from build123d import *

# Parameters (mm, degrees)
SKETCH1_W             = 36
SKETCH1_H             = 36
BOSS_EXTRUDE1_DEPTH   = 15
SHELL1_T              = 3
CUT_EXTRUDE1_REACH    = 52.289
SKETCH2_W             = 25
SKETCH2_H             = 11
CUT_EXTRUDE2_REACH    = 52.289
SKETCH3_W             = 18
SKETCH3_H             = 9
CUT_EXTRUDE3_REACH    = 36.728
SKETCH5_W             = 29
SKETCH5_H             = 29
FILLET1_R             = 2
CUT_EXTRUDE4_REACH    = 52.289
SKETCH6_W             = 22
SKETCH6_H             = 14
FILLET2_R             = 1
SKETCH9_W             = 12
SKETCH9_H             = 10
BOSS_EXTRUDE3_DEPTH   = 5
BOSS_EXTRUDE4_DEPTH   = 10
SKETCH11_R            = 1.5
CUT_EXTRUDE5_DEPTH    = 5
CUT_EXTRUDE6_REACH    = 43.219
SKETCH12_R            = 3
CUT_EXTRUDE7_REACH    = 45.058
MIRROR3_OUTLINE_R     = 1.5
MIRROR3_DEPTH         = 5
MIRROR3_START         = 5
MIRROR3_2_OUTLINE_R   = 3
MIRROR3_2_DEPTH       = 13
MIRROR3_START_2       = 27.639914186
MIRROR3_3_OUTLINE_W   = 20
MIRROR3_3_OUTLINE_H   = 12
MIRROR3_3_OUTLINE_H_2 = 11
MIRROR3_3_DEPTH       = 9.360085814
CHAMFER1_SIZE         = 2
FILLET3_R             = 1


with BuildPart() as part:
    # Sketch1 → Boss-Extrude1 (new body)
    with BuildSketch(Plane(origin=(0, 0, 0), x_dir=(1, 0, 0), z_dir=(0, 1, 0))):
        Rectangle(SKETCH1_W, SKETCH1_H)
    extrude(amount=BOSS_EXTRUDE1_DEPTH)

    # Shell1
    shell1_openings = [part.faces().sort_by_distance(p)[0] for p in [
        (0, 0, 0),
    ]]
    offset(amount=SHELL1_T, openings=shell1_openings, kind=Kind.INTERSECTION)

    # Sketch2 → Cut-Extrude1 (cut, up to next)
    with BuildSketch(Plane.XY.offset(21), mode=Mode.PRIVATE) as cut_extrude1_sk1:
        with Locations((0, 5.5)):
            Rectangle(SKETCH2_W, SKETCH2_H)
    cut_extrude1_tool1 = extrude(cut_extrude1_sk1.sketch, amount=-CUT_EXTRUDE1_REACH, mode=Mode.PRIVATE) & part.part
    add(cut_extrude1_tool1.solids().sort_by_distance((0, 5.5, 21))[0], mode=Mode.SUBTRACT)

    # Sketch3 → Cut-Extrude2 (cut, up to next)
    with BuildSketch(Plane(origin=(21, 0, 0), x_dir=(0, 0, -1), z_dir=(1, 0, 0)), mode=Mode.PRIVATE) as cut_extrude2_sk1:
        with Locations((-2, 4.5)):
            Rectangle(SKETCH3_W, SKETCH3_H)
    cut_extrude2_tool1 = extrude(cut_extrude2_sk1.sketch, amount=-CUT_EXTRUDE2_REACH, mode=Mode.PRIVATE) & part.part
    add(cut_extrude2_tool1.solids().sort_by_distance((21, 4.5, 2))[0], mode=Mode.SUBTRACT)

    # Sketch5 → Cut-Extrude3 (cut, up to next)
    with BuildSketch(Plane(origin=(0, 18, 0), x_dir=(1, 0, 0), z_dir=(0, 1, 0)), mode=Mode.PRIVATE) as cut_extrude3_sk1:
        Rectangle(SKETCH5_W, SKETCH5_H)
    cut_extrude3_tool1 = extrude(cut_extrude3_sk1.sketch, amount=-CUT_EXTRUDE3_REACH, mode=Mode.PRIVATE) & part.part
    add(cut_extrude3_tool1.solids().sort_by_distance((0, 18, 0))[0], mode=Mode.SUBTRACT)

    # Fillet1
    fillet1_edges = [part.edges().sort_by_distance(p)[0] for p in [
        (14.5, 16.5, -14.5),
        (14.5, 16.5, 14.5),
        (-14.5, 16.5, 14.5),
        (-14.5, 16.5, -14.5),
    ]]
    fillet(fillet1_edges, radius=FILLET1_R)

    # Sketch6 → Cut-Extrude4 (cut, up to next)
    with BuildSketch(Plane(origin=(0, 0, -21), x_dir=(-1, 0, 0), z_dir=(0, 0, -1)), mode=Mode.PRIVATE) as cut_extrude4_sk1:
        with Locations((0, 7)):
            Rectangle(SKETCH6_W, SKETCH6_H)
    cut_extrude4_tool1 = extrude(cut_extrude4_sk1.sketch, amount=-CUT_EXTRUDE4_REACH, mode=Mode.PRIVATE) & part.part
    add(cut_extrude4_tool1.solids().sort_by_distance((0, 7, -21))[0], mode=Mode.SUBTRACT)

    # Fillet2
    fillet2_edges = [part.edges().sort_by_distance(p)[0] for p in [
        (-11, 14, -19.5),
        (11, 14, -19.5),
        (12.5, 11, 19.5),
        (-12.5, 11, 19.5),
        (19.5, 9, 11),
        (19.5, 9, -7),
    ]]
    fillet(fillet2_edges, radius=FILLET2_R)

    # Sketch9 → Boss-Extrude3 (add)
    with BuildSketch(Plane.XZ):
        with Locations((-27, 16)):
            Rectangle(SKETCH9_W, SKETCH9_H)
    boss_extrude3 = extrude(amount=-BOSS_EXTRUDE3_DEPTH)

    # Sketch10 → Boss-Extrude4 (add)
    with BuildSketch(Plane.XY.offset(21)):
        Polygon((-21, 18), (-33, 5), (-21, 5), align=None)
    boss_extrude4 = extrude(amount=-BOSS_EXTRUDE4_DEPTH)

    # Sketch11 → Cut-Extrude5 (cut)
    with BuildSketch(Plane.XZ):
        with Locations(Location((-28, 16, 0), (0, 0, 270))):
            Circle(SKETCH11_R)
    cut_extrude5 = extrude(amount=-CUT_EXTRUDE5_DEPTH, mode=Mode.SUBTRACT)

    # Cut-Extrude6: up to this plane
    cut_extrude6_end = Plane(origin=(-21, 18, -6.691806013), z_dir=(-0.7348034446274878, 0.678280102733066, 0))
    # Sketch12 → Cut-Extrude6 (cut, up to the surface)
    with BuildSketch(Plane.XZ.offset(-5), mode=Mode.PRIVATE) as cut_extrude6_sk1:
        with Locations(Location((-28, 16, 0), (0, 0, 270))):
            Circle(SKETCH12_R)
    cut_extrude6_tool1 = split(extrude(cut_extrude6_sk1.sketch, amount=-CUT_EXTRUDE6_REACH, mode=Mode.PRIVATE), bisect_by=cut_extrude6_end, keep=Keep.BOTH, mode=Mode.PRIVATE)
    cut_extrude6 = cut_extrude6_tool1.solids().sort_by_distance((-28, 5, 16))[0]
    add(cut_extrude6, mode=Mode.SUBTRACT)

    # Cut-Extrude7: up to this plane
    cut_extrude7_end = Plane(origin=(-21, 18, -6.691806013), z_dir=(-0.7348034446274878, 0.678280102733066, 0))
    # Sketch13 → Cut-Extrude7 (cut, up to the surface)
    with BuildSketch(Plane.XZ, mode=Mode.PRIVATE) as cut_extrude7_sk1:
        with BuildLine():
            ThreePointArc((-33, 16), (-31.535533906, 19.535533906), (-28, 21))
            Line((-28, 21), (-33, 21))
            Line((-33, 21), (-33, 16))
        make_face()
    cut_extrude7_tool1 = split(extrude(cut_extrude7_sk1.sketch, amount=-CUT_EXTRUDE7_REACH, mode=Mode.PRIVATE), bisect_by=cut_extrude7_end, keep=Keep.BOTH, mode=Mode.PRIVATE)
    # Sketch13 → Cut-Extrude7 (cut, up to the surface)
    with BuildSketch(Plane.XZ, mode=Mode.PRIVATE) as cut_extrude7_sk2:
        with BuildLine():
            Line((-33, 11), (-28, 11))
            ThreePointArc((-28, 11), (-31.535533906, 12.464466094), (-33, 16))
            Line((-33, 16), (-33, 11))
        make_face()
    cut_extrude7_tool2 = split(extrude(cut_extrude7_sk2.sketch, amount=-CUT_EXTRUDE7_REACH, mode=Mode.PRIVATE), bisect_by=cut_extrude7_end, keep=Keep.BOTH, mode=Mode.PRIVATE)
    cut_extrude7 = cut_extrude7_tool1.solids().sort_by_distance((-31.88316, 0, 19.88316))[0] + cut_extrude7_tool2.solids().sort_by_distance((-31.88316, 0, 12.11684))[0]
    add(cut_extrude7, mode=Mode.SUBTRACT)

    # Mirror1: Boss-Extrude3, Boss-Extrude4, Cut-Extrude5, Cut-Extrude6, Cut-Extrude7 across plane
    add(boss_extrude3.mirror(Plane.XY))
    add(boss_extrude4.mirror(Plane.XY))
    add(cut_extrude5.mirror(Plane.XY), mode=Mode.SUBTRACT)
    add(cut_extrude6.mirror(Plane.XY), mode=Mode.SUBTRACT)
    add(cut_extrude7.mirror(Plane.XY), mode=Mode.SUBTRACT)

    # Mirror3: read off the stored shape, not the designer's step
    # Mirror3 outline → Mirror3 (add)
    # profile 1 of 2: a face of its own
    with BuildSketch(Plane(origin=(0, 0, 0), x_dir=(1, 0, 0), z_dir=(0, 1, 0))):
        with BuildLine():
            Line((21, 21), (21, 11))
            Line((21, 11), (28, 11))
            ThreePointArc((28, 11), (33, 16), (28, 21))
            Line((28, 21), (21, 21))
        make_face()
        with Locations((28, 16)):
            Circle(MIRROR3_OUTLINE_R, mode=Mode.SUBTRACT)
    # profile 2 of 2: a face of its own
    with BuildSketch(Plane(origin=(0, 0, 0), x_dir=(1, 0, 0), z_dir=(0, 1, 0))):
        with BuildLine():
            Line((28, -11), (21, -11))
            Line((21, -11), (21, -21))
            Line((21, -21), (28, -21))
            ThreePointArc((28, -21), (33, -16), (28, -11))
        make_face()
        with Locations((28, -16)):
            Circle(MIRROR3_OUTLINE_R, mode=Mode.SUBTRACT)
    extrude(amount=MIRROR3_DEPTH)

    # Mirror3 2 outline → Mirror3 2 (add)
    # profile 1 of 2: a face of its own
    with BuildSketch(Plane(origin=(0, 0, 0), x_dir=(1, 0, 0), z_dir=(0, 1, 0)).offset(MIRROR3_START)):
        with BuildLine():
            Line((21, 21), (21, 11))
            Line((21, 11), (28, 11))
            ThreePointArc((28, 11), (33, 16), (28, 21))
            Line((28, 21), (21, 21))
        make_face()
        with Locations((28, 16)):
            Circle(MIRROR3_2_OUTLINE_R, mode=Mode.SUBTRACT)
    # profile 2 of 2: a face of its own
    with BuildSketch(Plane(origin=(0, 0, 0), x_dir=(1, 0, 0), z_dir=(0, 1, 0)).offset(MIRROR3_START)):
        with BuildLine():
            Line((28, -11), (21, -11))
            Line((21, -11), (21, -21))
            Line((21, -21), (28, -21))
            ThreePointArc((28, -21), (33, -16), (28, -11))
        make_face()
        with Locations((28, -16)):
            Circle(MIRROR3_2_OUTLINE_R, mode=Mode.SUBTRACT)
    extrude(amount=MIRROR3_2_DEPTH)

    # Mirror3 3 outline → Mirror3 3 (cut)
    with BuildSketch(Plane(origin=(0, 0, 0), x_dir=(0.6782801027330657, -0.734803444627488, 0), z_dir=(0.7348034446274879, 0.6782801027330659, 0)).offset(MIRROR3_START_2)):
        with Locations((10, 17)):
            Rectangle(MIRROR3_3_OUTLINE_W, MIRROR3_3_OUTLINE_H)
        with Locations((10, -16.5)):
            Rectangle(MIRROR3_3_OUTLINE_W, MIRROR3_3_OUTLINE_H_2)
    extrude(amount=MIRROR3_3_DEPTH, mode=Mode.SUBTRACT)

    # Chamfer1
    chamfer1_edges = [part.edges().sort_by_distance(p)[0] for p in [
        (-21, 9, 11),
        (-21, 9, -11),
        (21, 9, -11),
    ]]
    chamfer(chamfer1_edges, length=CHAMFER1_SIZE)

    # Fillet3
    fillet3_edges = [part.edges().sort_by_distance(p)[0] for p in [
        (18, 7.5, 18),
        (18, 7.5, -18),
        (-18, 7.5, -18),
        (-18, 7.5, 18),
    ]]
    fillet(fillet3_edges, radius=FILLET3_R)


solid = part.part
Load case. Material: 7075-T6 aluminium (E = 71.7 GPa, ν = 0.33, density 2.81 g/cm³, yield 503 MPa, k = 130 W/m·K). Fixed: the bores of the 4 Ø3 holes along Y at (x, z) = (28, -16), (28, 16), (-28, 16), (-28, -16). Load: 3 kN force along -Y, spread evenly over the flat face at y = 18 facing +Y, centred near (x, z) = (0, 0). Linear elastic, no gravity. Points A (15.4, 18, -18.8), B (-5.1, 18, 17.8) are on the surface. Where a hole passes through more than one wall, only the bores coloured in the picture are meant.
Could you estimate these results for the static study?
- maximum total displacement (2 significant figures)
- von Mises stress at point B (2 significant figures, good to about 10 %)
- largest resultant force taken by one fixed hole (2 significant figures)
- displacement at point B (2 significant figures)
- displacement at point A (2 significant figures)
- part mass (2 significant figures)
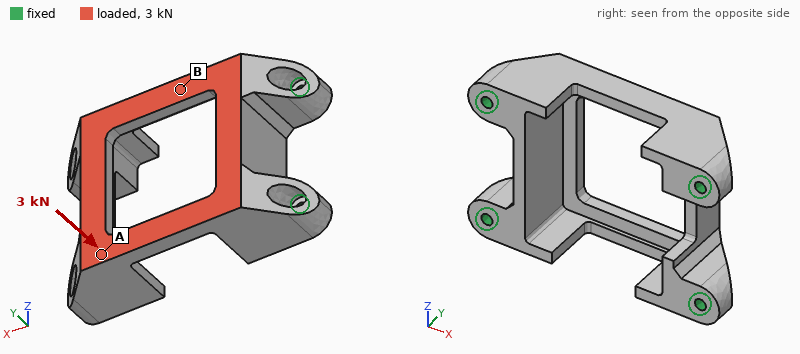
43 µm
45 MPa
960 N
23 µm
11 µm
34 g
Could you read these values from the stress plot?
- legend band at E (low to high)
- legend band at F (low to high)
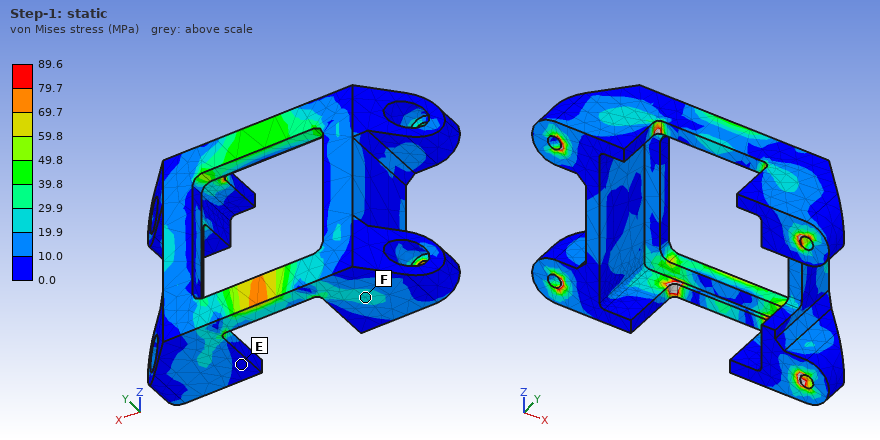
0.0 to 10.0 MPa
19.9 to 29.9 MPa
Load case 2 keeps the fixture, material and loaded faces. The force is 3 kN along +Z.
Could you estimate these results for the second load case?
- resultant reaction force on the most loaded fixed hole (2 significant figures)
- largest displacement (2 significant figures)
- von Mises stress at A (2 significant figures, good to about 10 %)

1.0 kN
61 µm
30 MPa
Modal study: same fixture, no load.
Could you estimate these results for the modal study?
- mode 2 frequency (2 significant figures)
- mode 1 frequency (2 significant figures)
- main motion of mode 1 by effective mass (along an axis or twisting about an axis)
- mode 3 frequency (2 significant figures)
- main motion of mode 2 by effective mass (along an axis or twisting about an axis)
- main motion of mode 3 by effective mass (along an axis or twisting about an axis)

11 kHz
10 kHz
along X
13 kHz
along Z
along Y
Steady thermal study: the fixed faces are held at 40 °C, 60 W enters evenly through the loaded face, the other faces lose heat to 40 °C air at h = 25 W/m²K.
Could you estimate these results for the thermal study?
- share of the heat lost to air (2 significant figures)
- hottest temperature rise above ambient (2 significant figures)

4.4 %
37 K
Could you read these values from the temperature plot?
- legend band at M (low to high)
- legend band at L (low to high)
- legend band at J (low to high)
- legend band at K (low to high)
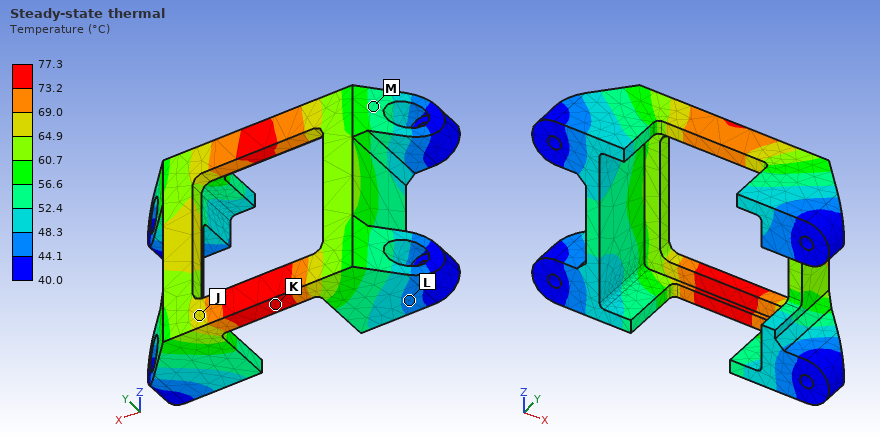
52.4 to 56.6 °C
44.1 to 48.3 °C
64.9 to 69.0 °C
73.2 to 77.3 °C
